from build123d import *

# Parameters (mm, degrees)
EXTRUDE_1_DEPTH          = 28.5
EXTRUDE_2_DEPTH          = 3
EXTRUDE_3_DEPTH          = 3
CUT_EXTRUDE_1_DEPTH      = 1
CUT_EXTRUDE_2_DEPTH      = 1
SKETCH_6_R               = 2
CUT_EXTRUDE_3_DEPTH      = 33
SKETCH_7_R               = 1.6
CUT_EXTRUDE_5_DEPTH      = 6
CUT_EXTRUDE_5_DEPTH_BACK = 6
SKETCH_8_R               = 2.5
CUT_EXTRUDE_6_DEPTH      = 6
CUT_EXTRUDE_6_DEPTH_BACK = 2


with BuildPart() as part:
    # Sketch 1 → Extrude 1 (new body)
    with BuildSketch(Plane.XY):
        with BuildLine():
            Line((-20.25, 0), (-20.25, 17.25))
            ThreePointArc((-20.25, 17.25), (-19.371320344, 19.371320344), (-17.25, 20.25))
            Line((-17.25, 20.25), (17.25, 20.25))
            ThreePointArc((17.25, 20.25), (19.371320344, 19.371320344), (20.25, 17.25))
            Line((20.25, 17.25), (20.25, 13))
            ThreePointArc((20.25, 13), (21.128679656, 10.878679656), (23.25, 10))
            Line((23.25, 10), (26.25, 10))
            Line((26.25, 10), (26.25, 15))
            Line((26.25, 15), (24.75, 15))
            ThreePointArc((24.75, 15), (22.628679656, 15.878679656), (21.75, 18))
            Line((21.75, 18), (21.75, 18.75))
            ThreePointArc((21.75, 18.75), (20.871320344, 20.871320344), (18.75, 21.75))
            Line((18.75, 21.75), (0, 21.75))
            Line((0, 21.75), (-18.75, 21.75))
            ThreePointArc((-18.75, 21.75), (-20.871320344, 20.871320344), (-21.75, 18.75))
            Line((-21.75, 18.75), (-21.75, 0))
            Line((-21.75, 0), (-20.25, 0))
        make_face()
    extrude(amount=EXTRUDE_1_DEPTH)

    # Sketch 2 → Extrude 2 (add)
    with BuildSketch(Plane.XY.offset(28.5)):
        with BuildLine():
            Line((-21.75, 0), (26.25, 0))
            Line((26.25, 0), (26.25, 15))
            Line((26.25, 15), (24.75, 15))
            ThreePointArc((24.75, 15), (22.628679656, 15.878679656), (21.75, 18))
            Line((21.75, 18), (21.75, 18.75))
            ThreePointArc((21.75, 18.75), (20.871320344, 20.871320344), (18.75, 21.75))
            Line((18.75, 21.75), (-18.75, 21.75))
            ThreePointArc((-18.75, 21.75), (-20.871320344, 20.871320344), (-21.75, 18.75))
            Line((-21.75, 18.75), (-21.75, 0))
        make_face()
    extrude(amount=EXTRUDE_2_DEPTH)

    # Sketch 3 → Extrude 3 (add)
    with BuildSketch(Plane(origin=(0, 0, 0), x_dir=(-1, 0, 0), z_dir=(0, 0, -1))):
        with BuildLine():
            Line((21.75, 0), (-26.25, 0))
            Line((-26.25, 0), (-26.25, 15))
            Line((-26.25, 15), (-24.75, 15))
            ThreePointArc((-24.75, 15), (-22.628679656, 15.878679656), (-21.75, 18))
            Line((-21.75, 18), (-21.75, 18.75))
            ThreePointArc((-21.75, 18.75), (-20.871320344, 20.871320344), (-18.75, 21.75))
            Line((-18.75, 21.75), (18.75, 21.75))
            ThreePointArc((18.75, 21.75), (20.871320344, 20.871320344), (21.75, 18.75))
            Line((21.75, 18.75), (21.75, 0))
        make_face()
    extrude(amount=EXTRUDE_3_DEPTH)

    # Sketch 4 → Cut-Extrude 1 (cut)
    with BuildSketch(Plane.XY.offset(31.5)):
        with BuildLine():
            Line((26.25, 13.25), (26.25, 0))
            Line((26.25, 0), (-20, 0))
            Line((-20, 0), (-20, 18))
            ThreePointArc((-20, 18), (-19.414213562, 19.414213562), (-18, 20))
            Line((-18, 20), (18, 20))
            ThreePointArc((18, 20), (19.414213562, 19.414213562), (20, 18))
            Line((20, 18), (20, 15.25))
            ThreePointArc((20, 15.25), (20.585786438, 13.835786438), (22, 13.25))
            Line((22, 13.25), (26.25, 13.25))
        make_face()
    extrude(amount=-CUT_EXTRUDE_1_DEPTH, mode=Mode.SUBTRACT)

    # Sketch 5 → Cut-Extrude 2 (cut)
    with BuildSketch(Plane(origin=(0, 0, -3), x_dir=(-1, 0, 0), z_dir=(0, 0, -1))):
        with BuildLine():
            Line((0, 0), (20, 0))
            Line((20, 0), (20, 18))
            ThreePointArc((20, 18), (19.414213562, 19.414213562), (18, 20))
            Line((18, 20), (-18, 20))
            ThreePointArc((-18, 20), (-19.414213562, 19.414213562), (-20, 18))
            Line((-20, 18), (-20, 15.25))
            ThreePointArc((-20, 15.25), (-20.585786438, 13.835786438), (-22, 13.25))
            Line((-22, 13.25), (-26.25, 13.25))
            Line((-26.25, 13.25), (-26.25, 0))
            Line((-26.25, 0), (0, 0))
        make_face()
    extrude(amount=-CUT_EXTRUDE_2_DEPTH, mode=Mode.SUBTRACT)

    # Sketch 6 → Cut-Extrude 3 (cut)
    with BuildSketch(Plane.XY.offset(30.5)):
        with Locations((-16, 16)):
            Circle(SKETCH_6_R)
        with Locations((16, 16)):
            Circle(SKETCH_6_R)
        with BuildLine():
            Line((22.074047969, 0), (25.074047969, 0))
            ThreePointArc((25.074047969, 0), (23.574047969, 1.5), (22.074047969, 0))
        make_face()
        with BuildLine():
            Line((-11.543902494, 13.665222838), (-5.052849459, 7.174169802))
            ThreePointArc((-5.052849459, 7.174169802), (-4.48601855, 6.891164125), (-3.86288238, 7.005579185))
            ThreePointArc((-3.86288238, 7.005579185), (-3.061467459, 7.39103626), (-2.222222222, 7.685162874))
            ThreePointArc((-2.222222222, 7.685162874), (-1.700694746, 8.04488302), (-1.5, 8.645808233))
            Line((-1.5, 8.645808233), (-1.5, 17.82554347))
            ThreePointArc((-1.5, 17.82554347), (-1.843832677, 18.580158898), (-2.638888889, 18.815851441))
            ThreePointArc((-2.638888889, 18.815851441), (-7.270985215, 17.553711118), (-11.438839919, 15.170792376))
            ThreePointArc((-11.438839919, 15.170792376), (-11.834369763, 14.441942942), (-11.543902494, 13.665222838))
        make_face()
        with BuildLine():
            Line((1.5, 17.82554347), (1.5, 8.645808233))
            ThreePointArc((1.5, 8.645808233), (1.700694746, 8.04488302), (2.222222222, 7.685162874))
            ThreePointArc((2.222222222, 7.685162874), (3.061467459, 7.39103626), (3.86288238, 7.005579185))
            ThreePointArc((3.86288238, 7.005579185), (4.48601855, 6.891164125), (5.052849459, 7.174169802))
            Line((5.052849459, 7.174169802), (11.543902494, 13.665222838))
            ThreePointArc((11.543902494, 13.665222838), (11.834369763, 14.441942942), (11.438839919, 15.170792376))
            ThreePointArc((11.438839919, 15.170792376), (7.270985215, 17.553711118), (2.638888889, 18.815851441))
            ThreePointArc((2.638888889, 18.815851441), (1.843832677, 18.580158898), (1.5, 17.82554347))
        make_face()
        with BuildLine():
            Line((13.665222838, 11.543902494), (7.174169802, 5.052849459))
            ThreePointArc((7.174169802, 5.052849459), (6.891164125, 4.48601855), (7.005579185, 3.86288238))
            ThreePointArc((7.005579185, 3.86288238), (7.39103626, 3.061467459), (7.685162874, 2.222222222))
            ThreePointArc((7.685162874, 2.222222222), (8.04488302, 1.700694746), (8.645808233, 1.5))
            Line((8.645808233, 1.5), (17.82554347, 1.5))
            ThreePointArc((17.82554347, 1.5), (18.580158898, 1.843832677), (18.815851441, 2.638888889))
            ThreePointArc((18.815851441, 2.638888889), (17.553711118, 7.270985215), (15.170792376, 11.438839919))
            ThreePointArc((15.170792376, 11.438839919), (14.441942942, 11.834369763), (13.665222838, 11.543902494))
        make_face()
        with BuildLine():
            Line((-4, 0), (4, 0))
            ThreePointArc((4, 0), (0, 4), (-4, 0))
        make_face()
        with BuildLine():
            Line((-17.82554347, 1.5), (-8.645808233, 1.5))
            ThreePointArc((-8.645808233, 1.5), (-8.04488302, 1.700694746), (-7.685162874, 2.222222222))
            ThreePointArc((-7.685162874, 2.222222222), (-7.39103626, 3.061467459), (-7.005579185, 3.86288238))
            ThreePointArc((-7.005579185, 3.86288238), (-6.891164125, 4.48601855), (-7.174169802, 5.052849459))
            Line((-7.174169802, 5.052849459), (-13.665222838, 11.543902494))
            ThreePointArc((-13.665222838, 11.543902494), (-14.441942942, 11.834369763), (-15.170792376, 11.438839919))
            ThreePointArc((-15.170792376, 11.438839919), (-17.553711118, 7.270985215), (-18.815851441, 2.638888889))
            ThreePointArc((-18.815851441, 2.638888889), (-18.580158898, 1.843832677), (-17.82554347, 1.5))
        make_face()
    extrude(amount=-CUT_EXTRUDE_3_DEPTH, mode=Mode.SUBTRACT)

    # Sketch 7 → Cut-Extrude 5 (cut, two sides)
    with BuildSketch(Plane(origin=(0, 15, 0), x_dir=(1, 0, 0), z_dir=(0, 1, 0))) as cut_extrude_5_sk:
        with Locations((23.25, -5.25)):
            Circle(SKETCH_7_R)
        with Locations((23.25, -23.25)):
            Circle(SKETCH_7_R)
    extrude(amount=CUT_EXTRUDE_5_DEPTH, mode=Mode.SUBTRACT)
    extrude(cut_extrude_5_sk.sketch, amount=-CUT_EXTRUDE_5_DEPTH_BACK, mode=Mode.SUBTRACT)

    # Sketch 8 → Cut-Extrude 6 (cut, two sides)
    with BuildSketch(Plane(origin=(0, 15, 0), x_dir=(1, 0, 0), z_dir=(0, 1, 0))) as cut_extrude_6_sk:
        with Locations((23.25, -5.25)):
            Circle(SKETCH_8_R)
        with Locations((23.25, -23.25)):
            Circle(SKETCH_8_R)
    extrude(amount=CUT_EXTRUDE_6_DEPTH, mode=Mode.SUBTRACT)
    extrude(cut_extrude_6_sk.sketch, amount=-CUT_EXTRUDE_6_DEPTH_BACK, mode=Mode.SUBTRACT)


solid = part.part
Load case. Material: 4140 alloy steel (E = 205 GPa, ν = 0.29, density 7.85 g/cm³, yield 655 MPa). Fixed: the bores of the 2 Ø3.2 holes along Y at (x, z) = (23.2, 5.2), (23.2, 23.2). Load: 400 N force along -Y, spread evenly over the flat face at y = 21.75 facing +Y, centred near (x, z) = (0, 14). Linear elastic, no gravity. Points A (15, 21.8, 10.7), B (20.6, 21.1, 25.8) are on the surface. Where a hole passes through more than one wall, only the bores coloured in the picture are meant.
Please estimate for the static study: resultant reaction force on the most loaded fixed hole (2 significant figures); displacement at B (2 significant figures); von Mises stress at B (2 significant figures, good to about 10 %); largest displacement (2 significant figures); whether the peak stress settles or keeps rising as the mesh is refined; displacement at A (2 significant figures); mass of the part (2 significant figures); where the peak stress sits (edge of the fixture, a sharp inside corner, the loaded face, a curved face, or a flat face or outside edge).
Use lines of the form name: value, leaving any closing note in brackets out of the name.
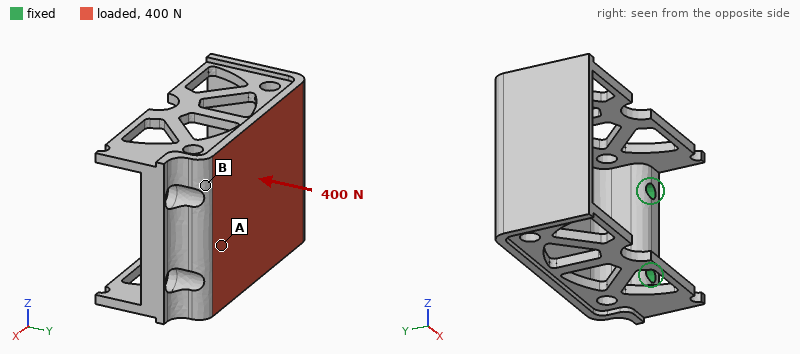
resultant reaction force on the most loaded fixed hole: 220 N
displacement at B: 0.024 mm
von Mises stress at B: 39 MPa
largest displacement: 0.15 mm
whether the peak stress settles or keeps rising as the mesh is refined: keeps rising
displacement at A: 0.038 mm
mass of the part: 50 g
where the peak stress sits: edge of the fixture
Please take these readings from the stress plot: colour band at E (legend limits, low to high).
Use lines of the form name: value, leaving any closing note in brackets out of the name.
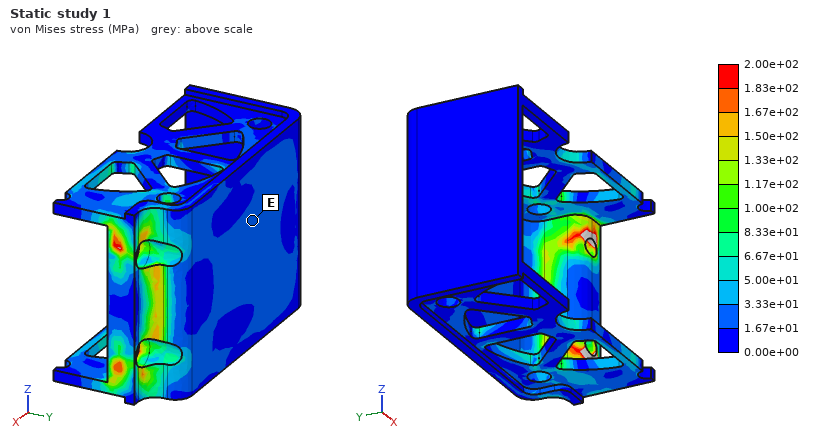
colour band at E: 1.67e+01 to 3.33e+01 MPa
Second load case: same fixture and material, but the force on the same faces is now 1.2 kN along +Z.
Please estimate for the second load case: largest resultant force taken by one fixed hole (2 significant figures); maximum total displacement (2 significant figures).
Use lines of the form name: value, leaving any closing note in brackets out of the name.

largest resultant force taken by one fixed hole: 1.4 kN
maximum total displacement: 0.25 mm
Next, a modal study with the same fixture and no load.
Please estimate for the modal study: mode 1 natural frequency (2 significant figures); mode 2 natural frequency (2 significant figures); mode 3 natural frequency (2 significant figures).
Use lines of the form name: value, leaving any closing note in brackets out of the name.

mode 1 natural frequency: 1300 Hz
mode 2 natural frequency: 1400 Hz
mode 3 natural frequency: 5000 Hz
